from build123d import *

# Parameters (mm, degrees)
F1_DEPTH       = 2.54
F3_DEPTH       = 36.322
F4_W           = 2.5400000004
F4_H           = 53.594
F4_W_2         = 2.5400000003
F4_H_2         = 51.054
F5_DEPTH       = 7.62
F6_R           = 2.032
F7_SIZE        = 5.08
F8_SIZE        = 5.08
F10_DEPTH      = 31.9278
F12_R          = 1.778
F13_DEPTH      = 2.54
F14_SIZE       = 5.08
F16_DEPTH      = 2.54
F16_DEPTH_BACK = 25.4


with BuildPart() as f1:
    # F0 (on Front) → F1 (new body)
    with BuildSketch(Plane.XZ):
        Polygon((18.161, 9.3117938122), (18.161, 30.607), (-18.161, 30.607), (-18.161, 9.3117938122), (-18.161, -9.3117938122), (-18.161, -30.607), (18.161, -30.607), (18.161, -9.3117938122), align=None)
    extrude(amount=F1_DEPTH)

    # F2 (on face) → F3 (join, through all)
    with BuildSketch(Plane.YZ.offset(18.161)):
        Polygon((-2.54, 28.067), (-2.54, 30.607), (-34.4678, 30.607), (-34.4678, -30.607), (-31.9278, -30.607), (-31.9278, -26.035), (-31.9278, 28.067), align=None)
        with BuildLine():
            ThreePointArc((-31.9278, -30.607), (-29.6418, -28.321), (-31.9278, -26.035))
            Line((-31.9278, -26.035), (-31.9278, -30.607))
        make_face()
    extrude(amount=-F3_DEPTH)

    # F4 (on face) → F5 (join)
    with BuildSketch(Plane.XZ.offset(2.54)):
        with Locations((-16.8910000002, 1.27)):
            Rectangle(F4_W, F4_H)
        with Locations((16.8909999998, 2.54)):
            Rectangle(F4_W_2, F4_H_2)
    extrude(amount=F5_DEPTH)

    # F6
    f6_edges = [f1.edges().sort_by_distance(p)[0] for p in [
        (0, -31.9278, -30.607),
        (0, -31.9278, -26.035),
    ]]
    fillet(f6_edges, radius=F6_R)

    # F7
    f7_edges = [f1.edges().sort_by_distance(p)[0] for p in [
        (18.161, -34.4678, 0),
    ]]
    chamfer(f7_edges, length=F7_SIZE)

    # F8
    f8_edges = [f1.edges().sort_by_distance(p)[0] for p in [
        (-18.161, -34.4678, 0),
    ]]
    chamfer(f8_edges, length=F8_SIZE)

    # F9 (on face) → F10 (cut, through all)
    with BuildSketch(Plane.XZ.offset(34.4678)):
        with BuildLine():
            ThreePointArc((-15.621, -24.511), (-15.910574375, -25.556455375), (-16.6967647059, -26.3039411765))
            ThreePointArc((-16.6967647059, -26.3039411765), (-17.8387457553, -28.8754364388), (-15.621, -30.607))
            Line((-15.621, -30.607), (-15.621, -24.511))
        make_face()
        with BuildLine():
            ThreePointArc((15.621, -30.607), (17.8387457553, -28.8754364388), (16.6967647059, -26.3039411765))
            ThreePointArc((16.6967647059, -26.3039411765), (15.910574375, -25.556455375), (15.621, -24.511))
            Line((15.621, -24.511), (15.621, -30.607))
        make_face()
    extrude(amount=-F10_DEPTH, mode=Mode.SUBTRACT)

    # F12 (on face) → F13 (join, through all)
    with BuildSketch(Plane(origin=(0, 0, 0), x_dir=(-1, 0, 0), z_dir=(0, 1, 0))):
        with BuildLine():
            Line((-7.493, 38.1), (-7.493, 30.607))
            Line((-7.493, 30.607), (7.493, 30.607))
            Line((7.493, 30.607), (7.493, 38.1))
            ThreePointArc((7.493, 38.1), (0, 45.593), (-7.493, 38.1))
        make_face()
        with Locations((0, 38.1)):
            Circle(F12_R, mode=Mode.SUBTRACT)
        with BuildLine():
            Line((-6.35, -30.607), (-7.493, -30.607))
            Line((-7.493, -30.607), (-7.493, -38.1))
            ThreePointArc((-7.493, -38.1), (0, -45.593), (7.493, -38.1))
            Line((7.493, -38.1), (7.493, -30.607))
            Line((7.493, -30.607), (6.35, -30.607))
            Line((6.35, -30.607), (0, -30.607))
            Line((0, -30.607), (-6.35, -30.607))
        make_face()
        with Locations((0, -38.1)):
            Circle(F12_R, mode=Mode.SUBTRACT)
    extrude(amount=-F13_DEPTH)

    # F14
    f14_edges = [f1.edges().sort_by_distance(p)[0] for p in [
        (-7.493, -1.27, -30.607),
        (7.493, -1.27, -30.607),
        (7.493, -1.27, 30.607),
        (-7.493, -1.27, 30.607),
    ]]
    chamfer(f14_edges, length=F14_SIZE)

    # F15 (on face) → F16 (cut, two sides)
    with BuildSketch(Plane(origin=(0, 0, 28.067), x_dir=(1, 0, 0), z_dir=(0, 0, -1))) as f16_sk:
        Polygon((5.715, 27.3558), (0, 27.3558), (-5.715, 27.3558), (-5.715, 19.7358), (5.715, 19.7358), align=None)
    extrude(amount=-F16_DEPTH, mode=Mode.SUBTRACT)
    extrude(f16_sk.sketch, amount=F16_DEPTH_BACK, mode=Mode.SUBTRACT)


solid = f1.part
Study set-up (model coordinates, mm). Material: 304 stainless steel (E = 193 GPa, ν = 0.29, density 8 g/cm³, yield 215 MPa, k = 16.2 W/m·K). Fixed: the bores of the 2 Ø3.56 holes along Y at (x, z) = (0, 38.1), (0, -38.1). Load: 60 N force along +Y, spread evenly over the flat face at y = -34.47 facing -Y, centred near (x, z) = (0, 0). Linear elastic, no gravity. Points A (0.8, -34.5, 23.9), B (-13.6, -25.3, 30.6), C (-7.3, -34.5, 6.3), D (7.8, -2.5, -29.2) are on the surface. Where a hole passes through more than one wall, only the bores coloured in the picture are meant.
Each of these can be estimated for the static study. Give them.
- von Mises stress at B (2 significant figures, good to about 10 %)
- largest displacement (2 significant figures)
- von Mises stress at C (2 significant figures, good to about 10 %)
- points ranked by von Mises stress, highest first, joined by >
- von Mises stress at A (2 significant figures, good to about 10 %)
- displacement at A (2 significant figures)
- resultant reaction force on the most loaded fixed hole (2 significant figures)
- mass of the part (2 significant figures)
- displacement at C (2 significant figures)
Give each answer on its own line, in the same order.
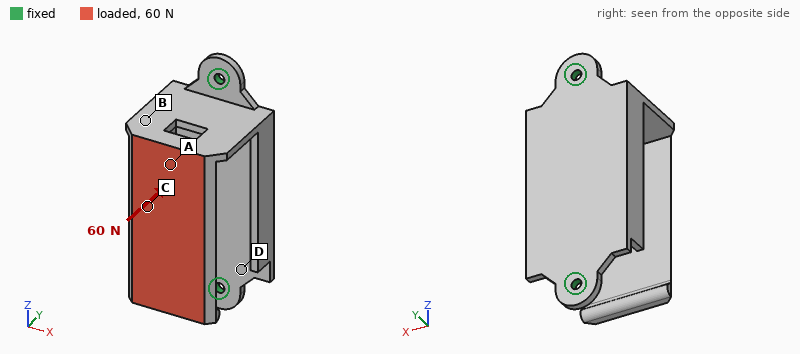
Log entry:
61 MPa
0.61 mm
22 MPa
B > A > C > D
41 MPa
0.11 mm
52 N
130 g
0.22 mm
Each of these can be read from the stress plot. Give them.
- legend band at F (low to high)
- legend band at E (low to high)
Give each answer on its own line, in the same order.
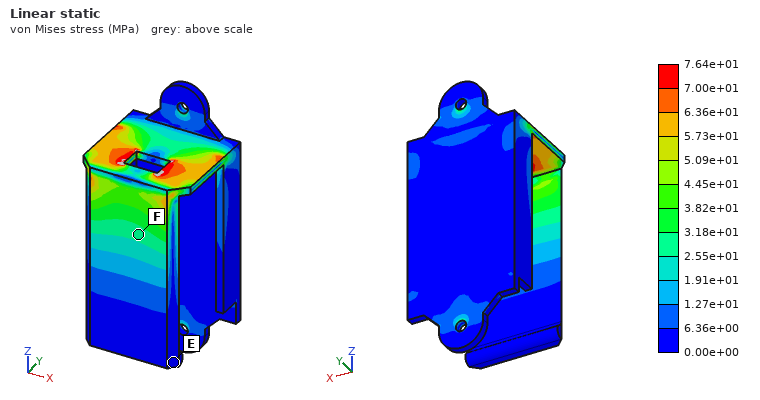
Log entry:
2.55e+01 to 3.18e+01 MPa
0.00e+00 to 6.36e+00 MPa
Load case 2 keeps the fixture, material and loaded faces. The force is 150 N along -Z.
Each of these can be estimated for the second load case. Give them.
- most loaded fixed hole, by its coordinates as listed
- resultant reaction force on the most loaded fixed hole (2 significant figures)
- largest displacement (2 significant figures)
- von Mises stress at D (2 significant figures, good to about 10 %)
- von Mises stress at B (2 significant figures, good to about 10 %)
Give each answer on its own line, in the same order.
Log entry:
(0, -38.1)
160 N
0.55 mm
12 MPa
53 MPa
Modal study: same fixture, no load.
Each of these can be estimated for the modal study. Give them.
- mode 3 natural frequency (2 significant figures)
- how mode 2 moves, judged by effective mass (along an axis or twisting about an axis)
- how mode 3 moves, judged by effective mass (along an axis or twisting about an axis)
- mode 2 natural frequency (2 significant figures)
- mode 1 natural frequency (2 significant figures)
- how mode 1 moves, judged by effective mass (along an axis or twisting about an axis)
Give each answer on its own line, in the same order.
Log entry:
1100 Hz
along X
along Z
520 Hz
290 Hz
along Y
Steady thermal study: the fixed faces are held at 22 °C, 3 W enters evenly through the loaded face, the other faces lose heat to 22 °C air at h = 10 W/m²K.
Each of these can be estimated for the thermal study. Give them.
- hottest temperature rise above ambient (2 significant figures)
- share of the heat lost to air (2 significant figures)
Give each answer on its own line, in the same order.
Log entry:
70 K
76 %
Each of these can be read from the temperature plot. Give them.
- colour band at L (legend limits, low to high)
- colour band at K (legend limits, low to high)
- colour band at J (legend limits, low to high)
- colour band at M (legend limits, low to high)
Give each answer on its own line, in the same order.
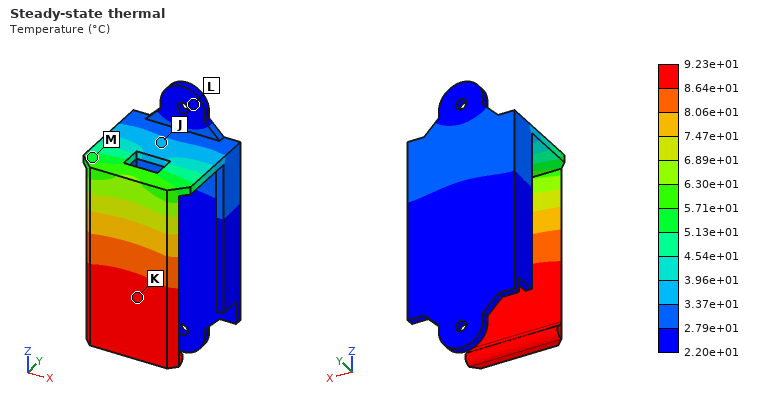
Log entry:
2.20e+01 to 2.79e+01 °C
8.64e+01 to 9.23e+01 °C
3.37e+01 to 3.96e+01 °C
5.13e+01 to 5.71e+01 °C
